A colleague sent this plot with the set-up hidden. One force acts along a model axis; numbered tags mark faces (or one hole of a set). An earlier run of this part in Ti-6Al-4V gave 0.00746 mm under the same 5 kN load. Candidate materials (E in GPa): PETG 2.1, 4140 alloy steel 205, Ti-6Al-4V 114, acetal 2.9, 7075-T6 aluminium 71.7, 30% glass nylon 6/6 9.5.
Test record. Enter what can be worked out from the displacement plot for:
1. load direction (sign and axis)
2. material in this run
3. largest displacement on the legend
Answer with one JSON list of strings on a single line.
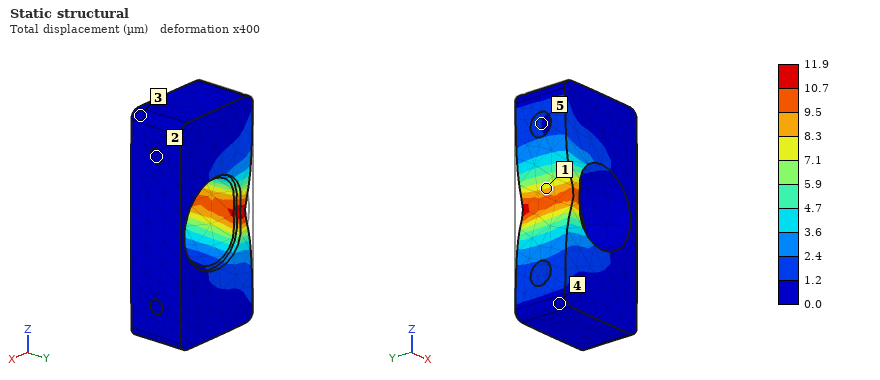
["+X", "7075-T6 aluminium", "11.9 µm"]
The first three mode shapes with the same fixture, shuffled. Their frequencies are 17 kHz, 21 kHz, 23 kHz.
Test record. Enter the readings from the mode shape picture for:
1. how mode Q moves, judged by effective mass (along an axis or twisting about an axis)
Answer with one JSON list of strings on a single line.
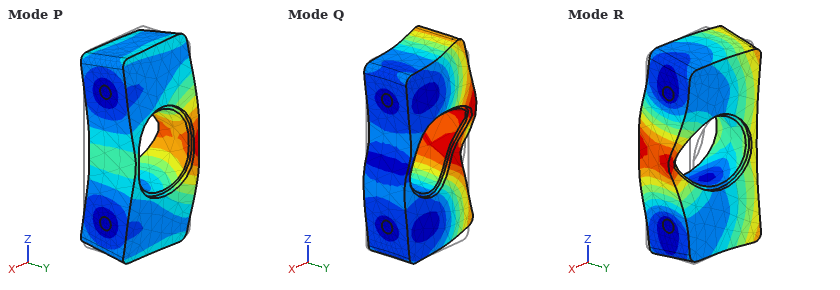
["along Z"]
